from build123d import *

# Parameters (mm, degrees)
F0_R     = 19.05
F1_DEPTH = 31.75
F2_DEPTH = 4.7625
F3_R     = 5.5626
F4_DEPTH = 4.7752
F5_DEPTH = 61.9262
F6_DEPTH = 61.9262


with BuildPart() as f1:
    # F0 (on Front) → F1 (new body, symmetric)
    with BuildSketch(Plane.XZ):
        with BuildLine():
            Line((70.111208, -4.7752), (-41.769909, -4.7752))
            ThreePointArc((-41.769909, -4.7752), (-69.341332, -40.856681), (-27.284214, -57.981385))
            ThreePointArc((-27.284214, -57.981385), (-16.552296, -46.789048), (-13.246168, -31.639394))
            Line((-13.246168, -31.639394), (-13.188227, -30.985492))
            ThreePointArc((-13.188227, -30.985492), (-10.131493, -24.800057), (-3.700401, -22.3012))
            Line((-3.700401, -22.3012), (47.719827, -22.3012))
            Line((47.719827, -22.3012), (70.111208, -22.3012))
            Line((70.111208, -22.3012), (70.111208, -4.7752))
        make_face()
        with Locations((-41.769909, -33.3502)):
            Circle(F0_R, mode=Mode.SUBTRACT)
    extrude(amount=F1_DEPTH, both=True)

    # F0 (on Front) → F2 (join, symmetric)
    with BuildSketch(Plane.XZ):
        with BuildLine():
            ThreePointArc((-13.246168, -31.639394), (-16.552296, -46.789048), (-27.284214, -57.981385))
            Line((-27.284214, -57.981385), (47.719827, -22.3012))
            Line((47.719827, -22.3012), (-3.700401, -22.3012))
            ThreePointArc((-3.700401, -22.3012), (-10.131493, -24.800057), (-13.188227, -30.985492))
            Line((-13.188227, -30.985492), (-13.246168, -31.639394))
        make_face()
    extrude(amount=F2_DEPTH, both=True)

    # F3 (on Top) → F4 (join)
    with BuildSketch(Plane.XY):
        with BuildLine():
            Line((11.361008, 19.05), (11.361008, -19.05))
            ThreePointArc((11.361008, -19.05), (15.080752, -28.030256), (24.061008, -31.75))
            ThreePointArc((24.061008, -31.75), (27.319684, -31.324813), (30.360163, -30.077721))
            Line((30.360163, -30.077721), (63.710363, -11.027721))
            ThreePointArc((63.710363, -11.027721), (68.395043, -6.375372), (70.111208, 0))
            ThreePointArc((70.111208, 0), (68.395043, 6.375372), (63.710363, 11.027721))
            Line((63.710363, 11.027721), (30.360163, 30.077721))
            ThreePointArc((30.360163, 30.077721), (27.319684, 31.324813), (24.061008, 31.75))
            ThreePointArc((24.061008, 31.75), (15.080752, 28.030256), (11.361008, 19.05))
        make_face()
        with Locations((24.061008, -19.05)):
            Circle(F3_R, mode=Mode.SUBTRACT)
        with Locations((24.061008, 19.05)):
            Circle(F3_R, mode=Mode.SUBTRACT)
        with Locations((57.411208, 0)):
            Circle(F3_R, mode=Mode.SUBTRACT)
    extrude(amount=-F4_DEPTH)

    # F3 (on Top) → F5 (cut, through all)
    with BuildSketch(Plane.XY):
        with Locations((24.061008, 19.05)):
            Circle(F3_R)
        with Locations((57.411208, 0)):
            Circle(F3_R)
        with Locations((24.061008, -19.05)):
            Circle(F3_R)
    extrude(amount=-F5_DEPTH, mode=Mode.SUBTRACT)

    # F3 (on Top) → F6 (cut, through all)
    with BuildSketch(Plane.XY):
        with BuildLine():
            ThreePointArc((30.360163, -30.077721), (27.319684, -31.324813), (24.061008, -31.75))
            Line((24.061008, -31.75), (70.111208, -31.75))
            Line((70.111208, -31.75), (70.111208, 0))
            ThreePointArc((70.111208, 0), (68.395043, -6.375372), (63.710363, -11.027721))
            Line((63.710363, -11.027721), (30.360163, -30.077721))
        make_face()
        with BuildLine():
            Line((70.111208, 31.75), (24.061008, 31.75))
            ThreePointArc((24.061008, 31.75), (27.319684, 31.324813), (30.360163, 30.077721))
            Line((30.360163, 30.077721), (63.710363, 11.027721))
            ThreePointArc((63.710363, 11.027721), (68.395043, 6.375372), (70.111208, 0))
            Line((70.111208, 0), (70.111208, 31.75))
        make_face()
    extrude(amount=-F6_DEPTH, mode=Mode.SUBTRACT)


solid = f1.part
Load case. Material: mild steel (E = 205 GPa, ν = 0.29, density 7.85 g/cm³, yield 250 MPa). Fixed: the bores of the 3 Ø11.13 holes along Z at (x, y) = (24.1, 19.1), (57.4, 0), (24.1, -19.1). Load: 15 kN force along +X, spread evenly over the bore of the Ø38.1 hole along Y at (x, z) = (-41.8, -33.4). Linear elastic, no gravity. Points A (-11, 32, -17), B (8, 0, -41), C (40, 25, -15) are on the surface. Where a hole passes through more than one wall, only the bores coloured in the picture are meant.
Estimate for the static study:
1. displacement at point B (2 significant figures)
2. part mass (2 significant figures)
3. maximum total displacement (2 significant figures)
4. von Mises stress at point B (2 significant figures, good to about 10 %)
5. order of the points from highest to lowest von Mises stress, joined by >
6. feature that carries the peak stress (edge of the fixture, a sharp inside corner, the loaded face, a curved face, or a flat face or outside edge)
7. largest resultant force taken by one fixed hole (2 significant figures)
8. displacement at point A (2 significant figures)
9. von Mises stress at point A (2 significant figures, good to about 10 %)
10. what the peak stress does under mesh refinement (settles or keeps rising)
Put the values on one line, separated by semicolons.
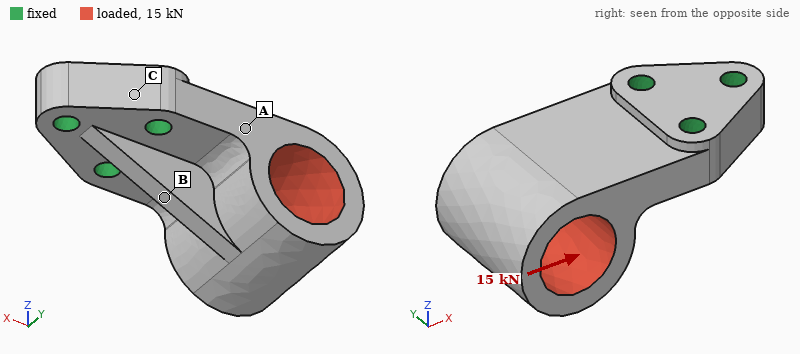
18 µm; 1.5 kg; 77 µm; 75 MPa; B > A > C; edge of the fixture; 6.1 kN; 14 µm; 22 MPa; keeps rising
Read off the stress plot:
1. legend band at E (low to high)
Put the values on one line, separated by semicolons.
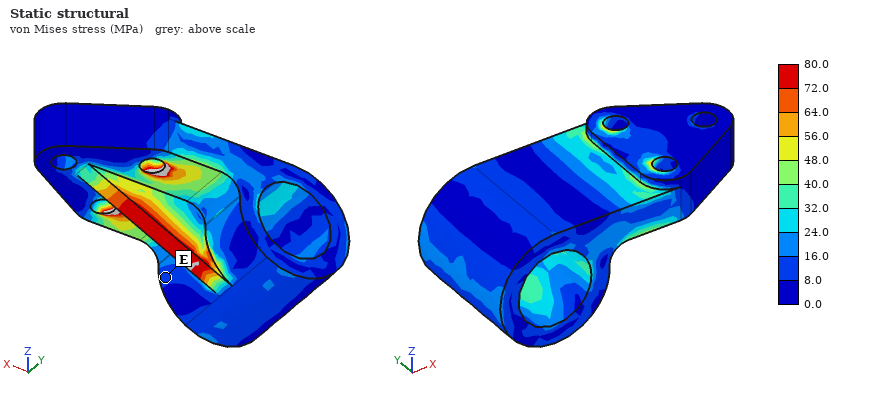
8.0 to 16.0 MPa
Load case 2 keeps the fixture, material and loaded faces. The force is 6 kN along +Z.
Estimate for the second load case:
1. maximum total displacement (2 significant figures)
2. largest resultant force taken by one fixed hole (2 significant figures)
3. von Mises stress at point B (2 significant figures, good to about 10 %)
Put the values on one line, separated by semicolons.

82 µm; 4.5 kN; 56 MPa
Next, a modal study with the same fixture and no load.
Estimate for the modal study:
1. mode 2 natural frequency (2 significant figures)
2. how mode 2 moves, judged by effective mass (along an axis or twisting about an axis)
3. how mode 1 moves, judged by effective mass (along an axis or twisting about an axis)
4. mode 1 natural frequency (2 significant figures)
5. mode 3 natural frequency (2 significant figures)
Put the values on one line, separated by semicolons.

3000 Hz; along Y; along Z; 1700 Hz; 5000 Hz
